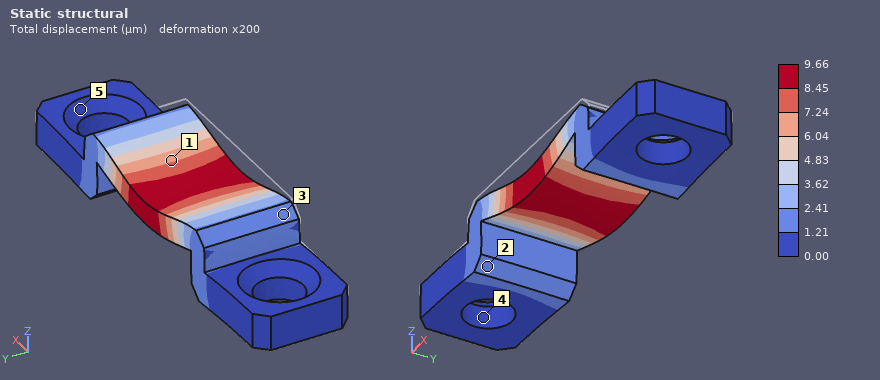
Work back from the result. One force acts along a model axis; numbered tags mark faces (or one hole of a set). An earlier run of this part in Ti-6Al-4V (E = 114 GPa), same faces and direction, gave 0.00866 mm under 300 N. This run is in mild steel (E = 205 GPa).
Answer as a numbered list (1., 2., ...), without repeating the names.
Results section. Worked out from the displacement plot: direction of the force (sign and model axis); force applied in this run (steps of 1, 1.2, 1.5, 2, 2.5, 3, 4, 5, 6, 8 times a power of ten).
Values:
1. -Z
2. 600 N
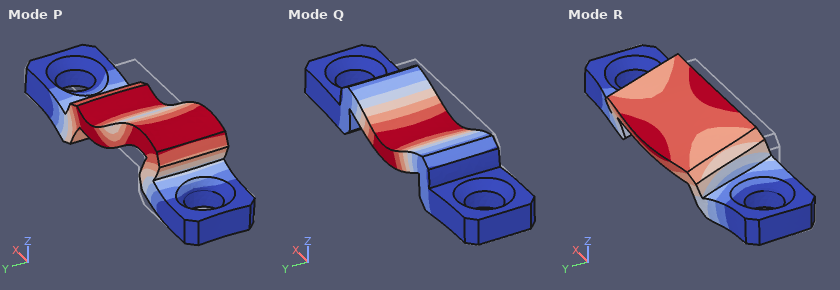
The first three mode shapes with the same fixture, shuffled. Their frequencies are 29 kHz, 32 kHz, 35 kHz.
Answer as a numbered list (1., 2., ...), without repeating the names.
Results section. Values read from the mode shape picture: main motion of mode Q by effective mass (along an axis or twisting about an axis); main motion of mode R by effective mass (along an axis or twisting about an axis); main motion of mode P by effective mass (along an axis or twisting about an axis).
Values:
1. along Z
2. along Y
3. along X
